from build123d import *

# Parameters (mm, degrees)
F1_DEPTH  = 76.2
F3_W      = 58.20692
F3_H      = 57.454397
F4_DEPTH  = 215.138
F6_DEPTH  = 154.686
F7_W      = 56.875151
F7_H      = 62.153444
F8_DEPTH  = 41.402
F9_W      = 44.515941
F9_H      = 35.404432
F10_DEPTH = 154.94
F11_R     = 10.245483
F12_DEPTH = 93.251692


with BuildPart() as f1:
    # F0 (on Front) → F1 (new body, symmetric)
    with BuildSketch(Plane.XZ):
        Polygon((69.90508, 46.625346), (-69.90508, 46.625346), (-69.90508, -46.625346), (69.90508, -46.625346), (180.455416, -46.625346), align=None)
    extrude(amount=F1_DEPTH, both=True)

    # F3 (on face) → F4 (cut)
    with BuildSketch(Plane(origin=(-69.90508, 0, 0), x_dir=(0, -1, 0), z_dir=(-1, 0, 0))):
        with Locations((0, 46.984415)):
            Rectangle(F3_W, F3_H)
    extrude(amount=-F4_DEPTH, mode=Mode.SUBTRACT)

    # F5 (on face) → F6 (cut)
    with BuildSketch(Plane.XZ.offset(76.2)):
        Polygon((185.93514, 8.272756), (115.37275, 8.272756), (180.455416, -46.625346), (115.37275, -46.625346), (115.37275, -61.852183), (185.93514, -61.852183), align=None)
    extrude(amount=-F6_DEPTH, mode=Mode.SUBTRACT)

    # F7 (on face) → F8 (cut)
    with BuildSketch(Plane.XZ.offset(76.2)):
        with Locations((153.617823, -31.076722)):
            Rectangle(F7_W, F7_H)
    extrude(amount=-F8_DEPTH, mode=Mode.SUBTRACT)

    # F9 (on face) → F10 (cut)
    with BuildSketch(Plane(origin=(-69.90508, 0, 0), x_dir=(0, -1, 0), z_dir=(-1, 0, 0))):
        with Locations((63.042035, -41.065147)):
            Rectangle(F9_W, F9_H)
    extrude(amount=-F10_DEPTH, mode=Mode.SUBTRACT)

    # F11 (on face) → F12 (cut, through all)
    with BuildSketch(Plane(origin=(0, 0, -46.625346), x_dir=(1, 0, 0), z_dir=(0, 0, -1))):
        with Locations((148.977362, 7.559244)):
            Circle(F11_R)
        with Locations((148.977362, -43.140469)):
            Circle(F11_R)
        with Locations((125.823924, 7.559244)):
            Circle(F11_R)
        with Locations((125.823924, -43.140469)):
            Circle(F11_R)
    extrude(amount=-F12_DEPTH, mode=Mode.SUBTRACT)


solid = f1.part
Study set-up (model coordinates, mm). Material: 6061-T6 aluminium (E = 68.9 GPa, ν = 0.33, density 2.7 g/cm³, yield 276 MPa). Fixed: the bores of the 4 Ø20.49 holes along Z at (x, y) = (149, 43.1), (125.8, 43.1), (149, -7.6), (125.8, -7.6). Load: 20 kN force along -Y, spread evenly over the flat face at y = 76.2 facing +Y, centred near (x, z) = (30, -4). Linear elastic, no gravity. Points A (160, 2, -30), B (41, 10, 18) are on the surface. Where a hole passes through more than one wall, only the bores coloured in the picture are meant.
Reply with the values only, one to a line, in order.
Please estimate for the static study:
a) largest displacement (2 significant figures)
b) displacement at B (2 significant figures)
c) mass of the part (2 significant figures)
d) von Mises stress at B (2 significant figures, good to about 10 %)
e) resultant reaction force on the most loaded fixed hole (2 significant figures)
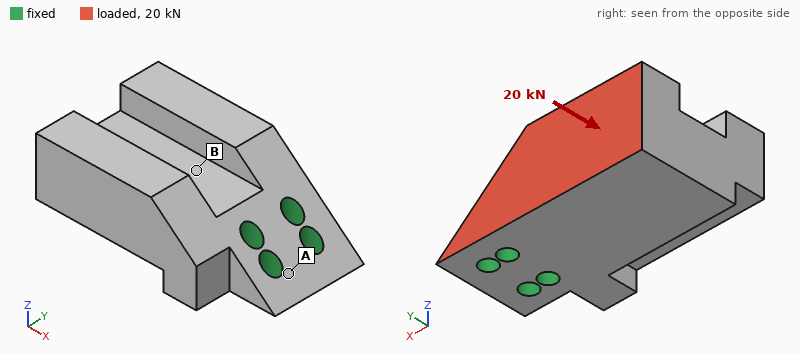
61 µm
23 µm
6.2 kg
4.8 MPa
27 kN
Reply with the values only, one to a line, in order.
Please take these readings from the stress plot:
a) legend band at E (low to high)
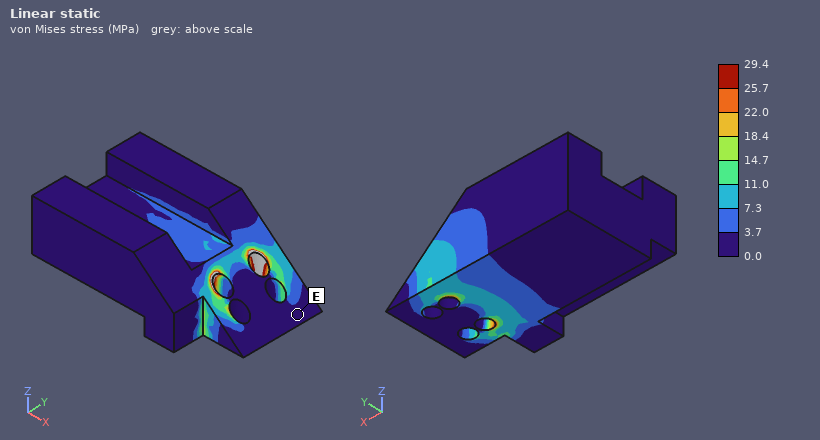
0.0 to 3.7 MPa
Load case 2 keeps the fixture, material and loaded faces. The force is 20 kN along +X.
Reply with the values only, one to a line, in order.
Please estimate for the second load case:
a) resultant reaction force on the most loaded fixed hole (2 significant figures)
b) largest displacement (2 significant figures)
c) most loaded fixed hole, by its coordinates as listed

24 kN
44 µm
(125.8, 43.1)
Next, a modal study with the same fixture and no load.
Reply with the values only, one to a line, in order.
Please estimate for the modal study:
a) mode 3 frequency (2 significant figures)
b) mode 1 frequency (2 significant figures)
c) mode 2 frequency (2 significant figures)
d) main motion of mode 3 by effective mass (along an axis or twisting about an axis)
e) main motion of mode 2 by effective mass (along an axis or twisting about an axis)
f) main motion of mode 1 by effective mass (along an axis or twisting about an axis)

2100 Hz
960 Hz
1400 Hz
twisting about X
along Y
along Z
